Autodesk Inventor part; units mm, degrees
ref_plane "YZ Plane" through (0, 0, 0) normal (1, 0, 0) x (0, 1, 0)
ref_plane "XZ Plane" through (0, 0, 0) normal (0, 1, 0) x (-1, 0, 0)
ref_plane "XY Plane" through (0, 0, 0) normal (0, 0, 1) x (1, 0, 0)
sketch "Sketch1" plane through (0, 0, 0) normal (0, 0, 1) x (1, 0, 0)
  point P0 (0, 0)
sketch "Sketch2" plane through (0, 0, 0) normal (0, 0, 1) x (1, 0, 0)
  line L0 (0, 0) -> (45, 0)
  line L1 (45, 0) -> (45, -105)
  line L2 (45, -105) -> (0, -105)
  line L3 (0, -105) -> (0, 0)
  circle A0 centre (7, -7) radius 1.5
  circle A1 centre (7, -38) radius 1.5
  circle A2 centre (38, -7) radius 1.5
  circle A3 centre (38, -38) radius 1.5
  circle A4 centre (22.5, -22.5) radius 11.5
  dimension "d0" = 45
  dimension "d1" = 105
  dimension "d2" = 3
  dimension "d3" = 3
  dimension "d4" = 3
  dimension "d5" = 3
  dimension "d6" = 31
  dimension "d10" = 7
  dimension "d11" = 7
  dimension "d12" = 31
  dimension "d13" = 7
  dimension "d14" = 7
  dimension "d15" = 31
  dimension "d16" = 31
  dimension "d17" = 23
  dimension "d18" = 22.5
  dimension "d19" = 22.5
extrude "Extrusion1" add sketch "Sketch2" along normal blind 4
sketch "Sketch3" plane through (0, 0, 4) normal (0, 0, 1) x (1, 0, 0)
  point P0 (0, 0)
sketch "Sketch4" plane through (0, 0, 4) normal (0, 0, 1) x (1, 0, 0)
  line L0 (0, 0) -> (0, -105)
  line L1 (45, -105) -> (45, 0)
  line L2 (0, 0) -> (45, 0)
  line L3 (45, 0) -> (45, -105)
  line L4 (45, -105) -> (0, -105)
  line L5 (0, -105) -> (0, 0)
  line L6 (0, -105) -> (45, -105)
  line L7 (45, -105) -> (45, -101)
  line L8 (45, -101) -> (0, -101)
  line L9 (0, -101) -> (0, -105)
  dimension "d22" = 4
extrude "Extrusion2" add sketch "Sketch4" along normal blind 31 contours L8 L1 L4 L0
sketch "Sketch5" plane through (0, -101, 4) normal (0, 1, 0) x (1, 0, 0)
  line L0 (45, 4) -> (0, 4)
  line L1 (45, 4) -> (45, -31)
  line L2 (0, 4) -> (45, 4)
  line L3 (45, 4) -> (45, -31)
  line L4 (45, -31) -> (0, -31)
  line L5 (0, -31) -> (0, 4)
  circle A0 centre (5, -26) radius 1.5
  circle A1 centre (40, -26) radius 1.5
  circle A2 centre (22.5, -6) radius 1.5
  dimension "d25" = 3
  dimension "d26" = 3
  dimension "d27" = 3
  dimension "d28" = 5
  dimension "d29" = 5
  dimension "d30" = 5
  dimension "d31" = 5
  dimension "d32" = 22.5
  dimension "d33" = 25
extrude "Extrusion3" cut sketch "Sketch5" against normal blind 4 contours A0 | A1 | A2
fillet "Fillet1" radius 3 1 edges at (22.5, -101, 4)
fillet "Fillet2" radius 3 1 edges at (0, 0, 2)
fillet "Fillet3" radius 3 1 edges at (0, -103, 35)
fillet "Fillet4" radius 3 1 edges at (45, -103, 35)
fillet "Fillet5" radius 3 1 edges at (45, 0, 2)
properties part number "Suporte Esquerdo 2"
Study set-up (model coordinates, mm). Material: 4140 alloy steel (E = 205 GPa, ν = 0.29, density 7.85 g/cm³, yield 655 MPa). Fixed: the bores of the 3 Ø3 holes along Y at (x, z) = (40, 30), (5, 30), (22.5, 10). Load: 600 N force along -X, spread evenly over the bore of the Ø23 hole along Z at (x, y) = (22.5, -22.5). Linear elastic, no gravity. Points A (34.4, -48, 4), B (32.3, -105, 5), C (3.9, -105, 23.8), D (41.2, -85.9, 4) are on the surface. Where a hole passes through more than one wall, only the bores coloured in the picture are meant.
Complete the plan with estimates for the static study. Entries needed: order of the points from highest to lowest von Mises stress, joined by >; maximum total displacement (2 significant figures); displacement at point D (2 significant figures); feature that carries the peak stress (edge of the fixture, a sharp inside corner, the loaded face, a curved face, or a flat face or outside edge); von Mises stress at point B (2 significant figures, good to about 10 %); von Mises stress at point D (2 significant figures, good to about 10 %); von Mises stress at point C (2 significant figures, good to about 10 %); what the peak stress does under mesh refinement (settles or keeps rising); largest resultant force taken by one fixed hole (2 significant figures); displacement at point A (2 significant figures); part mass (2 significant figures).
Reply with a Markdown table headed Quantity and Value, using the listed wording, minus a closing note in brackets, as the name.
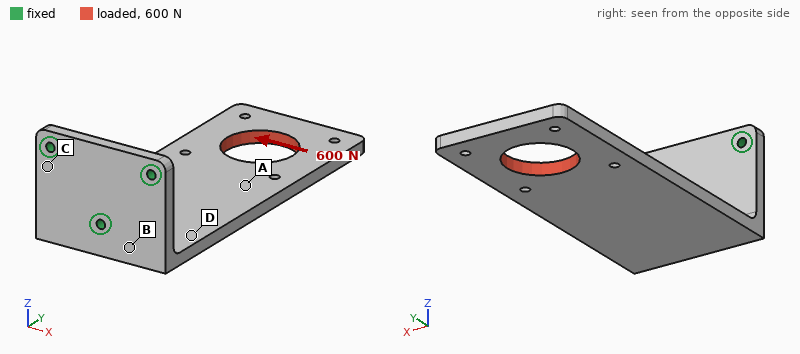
| Quantity | Value |
|---|---|
| order of the points from highest to lowest von Mises stress, joined by > | C > B > D > A |
| maximum total displacement | 0.59 mm |
| displacement at point D | 0.14 mm |
| feature that carries the peak stress | edge of the fixture |
| von Mises stress at point B | 110 MPa |
| von Mises stress at point D | 65 MPa |
| von Mises stress at point C | 160 MPa |
| what the peak stress does under mesh refinement | keeps rising |
| largest resultant force taken by one fixed hole | 670 N |
| displacement at point A | 0.31 mm |
| part mass | 180 g |
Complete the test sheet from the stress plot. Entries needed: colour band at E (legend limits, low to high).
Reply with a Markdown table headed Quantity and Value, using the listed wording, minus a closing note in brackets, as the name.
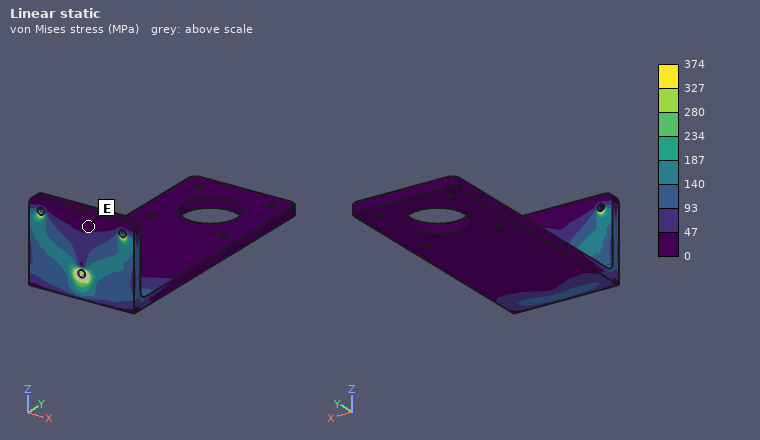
| Quantity | Value |
|---|---|
| colour band at E | 0 to 47 MPa |
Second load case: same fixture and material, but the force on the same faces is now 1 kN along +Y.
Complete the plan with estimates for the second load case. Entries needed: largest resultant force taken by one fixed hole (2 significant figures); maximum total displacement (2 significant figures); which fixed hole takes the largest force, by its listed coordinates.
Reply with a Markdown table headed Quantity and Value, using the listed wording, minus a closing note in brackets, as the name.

| Quantity | Value |
|---|---|
| largest resultant force taken by one fixed hole | 1.2 kN |
| maximum total displacement | 0.11 mm |
| which fixed hole takes the largest force, by its listed coordinates | (22.5, 10) |
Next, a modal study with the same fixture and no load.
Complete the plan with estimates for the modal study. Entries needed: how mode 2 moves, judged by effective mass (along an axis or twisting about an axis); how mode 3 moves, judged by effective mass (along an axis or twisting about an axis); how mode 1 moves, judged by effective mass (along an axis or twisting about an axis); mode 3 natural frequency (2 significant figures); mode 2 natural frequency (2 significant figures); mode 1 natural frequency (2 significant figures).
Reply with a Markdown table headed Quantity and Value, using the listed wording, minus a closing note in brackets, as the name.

| Quantity | Value |
|---|---|
| how mode 2 moves, judged by effective mass | along X |
| how mode 3 moves, judged by effective mass | twisting about Y |
| how mode 1 moves, judged by effective mass | along Z |
| mode 3 natural frequency | 1500 Hz |
| mode 2 natural frequency | 700 Hz |
| mode 1 natural frequency | 310 Hz |
